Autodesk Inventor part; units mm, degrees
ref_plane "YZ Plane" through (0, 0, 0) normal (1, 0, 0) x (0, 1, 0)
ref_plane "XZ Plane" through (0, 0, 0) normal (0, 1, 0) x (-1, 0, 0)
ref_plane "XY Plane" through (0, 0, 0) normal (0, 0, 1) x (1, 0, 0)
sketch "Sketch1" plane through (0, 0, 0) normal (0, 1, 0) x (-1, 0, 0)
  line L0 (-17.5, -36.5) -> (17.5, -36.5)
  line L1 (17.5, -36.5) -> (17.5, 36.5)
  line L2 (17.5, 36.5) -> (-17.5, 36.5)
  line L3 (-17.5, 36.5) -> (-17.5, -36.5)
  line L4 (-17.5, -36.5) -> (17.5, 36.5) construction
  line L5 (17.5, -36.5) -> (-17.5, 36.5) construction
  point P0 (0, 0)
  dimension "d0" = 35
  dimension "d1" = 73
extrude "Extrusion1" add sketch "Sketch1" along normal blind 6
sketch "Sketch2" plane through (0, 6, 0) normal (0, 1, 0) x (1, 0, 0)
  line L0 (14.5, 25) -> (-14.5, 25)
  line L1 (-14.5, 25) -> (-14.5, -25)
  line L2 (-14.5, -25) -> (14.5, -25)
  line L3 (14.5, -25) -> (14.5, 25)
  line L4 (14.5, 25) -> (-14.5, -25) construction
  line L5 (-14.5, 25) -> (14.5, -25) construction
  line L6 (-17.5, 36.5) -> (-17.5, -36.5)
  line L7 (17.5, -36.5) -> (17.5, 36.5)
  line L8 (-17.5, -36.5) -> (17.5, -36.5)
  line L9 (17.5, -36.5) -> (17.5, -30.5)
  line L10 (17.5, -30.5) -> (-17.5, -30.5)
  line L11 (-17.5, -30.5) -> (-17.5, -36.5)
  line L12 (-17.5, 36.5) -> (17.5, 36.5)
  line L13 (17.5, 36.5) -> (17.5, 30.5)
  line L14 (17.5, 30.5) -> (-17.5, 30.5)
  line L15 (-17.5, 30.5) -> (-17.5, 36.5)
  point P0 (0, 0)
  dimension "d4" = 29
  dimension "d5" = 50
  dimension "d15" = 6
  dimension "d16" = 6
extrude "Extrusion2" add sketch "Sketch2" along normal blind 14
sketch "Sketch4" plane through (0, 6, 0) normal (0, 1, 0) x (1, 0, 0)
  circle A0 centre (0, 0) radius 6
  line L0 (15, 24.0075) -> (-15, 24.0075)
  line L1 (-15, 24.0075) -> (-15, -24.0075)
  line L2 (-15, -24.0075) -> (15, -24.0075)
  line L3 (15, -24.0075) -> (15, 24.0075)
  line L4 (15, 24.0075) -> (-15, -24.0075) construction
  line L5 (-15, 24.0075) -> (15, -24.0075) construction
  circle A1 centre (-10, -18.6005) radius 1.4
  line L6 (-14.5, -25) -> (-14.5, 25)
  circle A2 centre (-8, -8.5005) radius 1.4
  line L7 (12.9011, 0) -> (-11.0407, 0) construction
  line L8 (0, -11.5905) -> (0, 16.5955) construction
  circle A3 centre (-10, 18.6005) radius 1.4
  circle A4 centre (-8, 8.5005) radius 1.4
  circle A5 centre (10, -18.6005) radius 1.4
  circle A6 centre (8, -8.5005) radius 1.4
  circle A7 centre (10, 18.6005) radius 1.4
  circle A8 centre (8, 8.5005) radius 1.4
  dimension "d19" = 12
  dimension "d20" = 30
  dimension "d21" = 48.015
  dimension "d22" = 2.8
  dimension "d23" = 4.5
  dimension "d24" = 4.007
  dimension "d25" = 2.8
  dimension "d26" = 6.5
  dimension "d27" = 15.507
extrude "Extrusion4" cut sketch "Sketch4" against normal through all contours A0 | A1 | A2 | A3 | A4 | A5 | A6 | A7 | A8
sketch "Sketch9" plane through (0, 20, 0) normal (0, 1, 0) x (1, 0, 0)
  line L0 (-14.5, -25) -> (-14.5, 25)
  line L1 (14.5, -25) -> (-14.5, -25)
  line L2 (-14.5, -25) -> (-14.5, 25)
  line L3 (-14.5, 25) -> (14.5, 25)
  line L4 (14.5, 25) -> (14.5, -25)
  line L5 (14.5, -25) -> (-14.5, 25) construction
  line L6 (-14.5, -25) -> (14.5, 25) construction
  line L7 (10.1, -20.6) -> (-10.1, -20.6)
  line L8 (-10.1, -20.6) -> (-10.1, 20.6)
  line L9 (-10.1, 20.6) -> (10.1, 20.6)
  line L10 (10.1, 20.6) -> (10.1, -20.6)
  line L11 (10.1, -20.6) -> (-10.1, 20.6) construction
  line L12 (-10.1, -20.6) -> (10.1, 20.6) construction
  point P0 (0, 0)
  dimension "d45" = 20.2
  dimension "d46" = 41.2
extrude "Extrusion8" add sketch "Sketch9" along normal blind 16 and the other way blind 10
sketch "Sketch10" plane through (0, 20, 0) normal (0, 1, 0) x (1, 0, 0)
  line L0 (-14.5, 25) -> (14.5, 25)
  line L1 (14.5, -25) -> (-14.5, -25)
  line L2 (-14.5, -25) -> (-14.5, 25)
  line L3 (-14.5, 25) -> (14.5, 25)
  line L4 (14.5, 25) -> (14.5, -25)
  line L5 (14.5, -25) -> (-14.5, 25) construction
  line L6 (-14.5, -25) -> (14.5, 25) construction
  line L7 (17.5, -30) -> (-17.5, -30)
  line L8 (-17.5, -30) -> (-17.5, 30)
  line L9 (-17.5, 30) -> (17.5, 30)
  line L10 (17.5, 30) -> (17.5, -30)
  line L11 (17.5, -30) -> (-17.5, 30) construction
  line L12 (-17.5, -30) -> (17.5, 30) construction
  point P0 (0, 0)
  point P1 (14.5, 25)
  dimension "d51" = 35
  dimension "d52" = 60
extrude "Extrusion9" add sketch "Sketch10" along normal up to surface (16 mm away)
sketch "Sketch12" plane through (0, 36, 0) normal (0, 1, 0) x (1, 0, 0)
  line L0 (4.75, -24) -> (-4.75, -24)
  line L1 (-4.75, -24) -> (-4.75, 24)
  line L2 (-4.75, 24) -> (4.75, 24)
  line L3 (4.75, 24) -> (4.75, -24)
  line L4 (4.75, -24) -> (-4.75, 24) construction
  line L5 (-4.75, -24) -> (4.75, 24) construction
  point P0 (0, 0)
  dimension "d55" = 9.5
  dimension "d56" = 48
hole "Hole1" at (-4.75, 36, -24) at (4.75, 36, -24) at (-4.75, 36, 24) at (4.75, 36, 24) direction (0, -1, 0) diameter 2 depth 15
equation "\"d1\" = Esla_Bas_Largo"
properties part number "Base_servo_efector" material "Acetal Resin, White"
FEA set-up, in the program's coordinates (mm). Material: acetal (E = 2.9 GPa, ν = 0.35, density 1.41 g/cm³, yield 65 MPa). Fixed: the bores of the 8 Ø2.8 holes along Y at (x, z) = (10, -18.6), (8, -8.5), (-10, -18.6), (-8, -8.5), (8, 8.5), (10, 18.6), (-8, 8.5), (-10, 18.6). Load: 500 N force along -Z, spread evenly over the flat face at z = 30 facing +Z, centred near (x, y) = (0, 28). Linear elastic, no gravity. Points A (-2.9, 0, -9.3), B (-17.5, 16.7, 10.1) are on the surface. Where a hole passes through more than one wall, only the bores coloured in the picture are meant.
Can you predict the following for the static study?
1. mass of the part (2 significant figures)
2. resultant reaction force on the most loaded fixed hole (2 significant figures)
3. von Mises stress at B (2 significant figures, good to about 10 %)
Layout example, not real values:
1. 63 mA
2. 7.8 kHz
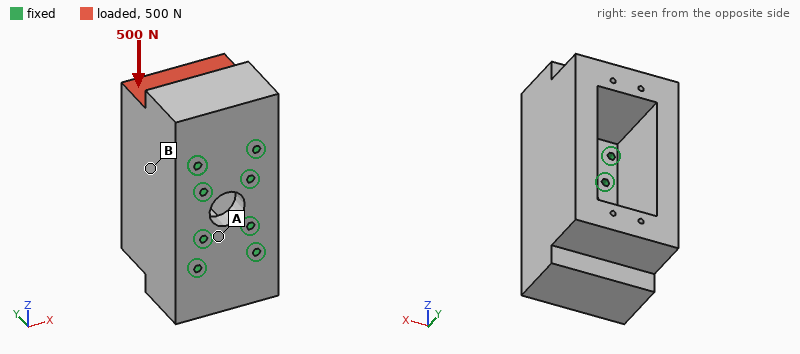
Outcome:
1. 79 g
2. 160 N
3. 1.7 MPa
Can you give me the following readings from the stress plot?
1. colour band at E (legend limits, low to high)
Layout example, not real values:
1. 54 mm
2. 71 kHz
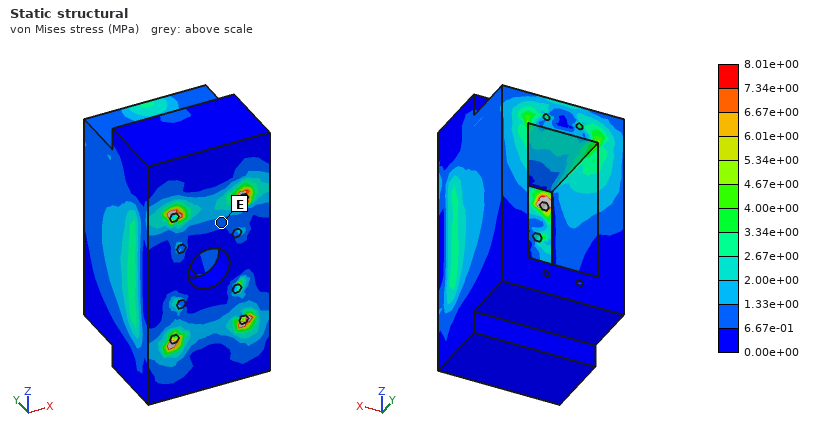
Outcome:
1. 6.67e-01 to 1.33e+00 MPa
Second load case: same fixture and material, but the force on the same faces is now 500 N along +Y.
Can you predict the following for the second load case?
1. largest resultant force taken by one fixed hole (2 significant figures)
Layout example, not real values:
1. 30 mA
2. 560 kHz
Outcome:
1. 280 N
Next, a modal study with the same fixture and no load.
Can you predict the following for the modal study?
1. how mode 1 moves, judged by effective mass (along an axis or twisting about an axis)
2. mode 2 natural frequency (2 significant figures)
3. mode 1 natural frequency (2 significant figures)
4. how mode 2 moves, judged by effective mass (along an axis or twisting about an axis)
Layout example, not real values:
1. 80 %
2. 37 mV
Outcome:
1. along X
2. 2100 Hz
3. 1900 Hz
4. along Z
